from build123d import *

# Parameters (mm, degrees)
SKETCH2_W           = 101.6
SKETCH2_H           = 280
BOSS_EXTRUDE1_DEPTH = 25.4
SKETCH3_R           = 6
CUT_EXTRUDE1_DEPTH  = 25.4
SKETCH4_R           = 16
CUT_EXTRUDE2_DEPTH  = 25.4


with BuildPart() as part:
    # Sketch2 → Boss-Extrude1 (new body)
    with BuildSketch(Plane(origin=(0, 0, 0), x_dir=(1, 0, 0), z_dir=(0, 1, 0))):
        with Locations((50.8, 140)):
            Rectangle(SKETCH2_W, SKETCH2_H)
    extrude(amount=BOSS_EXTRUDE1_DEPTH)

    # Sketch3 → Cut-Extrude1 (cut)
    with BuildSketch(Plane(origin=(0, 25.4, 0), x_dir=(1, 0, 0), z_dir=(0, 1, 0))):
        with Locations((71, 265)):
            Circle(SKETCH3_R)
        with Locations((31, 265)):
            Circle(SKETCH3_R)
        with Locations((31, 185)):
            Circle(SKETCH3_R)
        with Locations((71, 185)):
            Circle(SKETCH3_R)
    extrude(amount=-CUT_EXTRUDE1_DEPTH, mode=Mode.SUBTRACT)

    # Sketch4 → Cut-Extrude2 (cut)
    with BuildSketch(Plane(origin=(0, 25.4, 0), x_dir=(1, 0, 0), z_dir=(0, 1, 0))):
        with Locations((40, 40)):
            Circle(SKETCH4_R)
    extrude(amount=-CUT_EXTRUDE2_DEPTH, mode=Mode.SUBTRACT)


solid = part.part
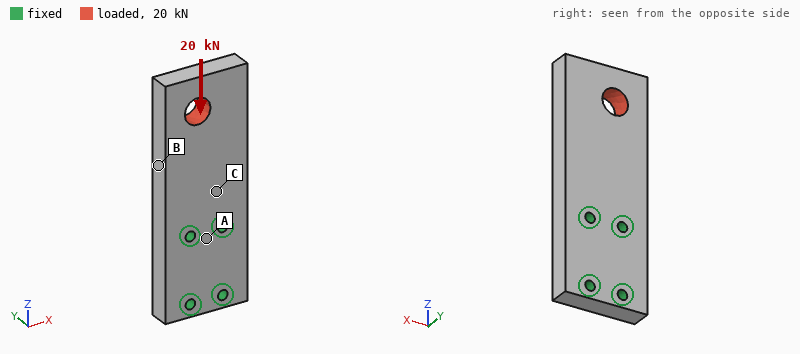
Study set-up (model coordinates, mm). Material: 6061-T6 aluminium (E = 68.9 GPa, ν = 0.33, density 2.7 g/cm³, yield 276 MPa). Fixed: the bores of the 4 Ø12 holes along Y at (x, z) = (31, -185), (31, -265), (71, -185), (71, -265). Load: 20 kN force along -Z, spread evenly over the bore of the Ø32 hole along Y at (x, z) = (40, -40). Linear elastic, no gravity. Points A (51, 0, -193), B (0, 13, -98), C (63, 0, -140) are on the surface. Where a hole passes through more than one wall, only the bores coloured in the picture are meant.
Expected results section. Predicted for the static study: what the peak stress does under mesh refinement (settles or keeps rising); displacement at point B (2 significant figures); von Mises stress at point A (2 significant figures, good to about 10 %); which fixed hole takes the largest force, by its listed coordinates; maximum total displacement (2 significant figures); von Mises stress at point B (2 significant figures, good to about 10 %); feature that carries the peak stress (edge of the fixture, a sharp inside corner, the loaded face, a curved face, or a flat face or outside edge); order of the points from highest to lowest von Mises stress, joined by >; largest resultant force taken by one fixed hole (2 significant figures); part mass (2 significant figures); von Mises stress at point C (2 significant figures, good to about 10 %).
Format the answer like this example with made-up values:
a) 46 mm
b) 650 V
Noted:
a) keeps rising
b) 21 µm
c) 3.0 MPa
d) (31, -185)
e) 38 µm
f) 13 MPa
g) edge of the fixture
h) B > C > A
i) 12 kN
j) 1.9 kg
k) 7.1 MPa
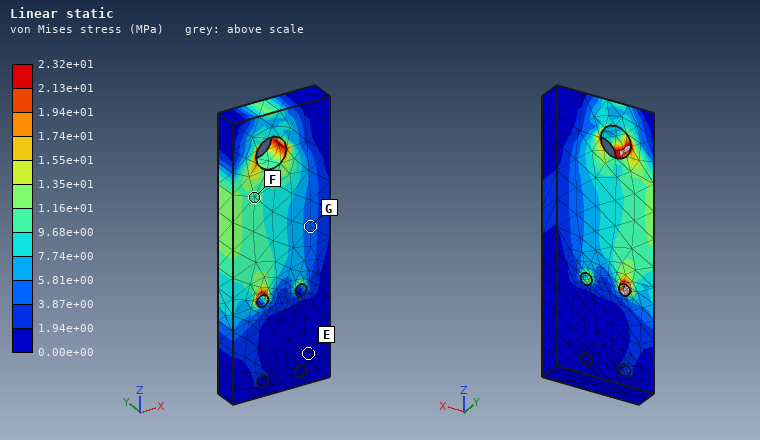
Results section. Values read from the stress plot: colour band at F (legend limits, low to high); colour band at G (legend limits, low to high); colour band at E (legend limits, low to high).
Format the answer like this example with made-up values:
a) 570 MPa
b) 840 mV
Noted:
a) 9.68e+00 to 1.16e+01 MPa
b) 3.87e+00 to 5.81e+00 MPa
c) 0.00e+00 to 1.94e+00 MPa
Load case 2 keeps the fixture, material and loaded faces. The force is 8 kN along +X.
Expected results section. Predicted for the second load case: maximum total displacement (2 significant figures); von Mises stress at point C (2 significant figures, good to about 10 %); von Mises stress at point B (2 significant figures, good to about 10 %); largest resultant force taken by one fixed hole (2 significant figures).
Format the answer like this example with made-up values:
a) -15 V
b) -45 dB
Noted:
a) 0.13 mm
b) 10 MPa
c) 11 MPa
d) 17 kN
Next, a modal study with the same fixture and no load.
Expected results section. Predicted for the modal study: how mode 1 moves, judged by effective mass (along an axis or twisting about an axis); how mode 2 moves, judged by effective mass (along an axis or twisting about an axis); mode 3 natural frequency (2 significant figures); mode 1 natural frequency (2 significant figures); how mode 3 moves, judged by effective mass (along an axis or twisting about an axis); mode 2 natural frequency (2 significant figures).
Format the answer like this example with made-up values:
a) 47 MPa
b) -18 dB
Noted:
a) along Y
b) along X
c) 2000 Hz
d) 620 Hz
e) twisting about Z
f) 1800 Hz
